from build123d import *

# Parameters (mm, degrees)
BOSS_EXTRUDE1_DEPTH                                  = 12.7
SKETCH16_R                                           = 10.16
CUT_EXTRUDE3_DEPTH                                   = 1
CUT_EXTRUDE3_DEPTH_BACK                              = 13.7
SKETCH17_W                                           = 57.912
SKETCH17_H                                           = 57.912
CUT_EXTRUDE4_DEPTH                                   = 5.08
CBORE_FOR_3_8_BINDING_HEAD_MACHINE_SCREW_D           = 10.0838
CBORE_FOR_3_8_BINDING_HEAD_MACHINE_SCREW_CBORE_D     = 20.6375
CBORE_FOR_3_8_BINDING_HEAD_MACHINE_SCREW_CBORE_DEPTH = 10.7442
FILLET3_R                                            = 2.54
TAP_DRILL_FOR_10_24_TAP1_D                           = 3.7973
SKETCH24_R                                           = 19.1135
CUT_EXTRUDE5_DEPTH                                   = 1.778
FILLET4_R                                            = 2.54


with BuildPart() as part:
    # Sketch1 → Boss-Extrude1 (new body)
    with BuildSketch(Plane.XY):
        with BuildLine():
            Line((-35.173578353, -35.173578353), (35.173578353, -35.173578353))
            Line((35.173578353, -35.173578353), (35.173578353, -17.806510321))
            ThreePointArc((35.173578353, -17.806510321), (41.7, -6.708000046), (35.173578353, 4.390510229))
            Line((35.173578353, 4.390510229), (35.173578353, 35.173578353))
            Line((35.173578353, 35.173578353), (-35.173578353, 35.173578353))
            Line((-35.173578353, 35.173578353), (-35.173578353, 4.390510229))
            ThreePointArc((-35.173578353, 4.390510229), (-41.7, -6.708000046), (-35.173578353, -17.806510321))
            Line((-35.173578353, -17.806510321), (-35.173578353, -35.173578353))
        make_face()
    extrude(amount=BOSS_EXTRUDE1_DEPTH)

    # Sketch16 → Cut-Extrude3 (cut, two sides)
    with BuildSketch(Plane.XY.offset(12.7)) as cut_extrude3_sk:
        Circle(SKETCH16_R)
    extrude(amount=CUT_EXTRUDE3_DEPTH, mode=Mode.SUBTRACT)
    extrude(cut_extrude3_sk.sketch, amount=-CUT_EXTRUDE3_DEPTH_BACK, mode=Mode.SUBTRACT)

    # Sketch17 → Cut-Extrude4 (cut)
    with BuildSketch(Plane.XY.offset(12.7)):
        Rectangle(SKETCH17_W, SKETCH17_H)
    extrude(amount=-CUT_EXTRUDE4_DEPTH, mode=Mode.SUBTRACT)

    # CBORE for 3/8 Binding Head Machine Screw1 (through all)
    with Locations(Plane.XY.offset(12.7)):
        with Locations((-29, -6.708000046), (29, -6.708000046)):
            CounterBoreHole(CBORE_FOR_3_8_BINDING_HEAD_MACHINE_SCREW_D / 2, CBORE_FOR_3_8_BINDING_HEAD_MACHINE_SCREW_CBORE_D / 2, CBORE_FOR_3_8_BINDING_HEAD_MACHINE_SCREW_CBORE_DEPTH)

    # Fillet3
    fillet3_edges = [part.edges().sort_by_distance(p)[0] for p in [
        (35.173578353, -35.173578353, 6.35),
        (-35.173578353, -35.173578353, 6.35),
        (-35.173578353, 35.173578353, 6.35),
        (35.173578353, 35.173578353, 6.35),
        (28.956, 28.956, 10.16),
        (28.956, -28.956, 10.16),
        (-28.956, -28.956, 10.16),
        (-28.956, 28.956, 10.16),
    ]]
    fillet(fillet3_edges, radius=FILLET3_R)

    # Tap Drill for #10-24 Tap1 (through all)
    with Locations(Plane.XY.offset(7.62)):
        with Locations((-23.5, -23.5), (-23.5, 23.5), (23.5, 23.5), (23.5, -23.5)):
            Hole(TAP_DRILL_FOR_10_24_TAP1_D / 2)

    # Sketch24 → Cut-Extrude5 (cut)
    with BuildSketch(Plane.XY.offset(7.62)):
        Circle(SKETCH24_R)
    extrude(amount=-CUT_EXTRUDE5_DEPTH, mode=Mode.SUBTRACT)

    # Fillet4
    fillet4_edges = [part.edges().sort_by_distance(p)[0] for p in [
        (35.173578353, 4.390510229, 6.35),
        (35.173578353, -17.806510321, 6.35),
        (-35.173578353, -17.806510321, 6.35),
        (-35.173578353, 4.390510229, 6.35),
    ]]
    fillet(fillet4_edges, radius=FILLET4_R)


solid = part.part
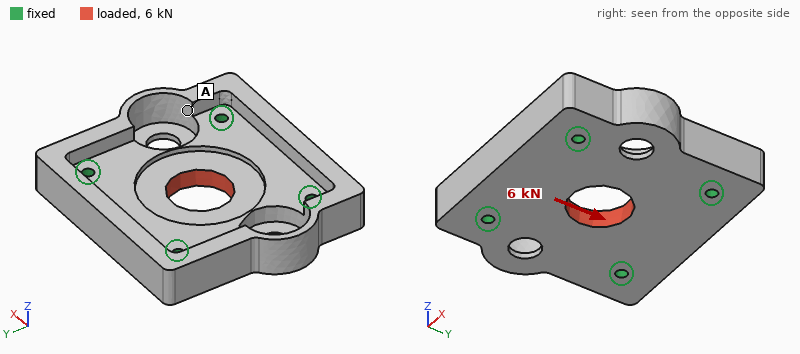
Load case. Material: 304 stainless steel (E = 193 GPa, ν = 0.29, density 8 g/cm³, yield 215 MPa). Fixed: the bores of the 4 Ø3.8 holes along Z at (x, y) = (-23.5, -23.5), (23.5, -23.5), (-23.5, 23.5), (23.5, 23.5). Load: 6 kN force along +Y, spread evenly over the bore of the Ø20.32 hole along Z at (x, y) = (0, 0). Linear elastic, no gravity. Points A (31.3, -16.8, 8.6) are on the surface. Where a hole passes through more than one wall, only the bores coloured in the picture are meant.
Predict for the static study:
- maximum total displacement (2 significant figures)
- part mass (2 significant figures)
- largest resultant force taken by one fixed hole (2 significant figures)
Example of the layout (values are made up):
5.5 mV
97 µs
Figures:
3.1 µm
310 g
1.7 kN
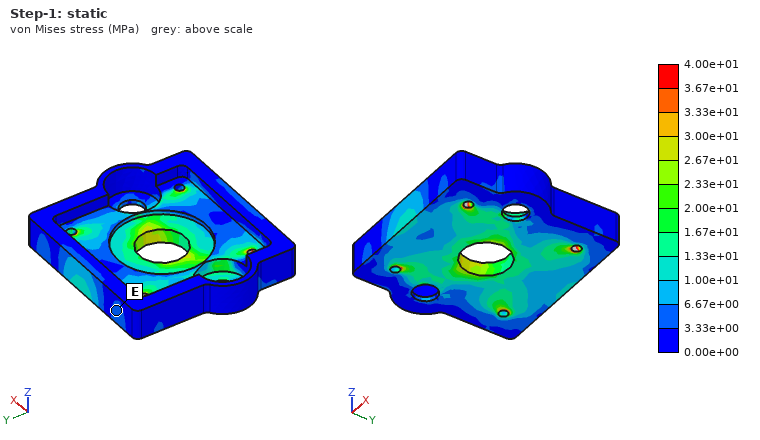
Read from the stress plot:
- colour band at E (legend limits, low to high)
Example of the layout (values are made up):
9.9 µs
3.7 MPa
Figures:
3.33e+00 to 6.67e+00 MPa
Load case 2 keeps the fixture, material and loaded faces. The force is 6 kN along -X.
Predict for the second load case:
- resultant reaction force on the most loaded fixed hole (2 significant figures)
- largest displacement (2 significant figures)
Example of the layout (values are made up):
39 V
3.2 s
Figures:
1.8 kN
3.1 µm
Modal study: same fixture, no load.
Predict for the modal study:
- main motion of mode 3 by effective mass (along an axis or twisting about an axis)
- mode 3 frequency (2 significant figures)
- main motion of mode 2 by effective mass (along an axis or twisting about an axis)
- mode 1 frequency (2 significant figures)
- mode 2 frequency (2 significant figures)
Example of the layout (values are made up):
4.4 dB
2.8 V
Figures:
twisting about Y
12 kHz
along Z
11 kHz
12 kHz
